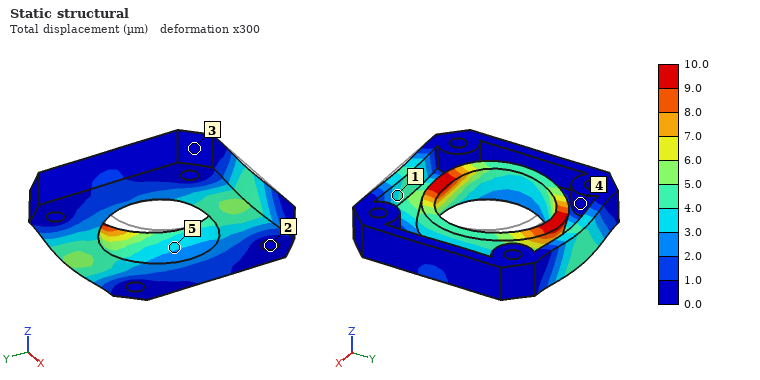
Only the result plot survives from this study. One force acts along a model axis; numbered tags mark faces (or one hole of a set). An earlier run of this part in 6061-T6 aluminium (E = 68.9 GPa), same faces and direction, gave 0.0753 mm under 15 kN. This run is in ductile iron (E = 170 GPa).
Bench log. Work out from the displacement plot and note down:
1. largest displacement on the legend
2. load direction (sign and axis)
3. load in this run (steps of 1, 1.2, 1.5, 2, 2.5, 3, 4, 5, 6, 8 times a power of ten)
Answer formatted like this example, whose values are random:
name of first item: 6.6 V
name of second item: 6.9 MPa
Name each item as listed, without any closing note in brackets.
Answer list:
largest displacement on the legend: 10.0 µm
load direction: +Y
load in this run: 5 kN
